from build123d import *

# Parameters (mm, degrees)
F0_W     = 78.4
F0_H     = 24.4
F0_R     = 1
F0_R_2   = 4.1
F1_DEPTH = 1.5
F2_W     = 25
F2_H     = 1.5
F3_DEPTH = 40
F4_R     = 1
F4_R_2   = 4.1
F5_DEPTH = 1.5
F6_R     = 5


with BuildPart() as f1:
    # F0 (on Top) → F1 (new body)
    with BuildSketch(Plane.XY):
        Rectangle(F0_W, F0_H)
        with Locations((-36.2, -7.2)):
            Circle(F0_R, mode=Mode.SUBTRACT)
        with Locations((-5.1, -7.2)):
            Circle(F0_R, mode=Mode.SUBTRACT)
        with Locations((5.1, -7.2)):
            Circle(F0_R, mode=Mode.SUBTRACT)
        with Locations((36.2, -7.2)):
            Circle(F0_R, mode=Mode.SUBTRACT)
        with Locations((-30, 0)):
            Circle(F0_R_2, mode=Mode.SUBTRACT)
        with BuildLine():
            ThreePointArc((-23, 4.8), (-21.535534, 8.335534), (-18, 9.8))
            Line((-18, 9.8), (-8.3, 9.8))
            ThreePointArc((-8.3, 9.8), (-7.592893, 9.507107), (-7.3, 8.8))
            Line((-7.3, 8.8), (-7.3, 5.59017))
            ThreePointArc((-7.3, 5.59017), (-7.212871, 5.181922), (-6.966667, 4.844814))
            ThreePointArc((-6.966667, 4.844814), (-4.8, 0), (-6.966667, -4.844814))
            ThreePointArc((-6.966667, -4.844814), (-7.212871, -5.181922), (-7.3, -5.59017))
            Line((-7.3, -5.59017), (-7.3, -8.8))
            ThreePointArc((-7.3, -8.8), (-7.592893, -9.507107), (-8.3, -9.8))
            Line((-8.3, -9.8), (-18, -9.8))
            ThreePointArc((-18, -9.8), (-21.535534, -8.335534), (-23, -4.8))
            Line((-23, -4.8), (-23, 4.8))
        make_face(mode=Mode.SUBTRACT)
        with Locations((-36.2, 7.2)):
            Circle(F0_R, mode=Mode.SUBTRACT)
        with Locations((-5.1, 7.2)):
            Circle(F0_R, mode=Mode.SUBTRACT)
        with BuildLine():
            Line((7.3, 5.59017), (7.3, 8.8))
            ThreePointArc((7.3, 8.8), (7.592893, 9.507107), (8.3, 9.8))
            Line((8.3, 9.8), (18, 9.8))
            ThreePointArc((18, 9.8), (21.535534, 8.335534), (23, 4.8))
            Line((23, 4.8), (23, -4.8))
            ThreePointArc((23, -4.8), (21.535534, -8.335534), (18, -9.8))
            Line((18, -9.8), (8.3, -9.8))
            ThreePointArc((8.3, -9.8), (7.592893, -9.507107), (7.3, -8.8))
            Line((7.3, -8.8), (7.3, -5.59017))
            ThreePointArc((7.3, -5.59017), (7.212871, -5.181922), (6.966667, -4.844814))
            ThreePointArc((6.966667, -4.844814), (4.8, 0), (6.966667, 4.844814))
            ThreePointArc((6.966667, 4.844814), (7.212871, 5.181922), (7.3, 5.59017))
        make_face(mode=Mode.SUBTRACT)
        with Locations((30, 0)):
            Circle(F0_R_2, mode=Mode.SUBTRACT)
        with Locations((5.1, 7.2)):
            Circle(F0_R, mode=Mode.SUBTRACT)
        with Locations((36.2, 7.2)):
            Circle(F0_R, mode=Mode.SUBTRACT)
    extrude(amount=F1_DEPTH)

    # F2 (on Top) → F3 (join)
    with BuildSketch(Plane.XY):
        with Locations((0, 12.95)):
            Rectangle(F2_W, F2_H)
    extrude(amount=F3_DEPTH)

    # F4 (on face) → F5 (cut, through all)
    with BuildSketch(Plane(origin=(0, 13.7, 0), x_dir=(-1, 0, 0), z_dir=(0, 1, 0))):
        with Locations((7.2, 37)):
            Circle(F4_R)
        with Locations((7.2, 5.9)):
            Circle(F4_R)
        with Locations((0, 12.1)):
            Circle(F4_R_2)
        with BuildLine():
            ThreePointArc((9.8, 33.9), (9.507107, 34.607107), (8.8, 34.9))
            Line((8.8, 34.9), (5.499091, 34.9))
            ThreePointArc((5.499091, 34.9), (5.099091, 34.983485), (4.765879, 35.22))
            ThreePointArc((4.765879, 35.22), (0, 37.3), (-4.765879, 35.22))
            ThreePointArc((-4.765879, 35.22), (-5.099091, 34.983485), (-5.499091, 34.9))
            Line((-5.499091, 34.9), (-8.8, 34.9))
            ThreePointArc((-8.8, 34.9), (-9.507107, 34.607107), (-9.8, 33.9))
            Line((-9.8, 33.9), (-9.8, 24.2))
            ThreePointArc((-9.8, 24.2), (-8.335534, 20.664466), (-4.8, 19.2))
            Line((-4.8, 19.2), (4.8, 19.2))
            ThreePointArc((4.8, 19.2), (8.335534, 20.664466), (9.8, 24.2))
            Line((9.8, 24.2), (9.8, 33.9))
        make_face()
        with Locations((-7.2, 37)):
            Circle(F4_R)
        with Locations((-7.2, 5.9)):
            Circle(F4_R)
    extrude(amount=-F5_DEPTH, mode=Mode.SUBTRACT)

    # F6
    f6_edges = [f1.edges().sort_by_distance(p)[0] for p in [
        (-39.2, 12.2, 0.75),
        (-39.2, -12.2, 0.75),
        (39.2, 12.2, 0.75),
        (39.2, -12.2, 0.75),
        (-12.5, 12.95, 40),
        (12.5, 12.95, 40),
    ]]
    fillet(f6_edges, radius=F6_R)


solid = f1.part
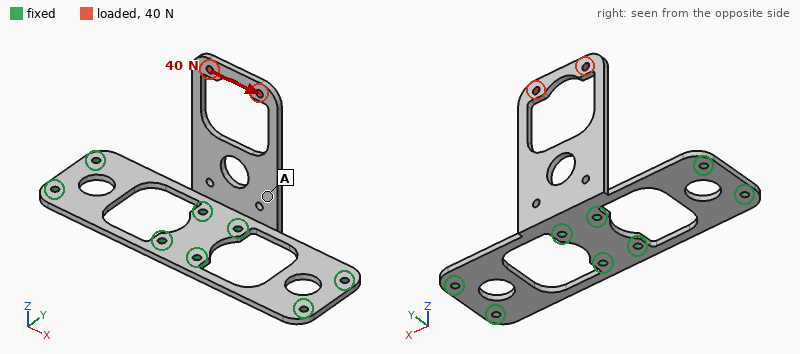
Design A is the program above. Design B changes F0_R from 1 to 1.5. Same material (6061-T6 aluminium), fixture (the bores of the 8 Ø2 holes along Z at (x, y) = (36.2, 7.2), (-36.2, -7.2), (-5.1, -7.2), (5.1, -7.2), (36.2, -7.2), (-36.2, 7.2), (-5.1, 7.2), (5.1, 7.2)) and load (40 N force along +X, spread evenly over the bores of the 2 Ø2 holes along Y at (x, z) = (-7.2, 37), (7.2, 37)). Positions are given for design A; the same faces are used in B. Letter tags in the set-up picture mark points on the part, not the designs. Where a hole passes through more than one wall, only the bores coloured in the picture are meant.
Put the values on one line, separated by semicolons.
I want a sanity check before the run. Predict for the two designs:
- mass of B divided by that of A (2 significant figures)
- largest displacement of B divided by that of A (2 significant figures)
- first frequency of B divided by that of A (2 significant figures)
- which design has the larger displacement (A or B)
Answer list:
0.98; 0.85; 1.0; A
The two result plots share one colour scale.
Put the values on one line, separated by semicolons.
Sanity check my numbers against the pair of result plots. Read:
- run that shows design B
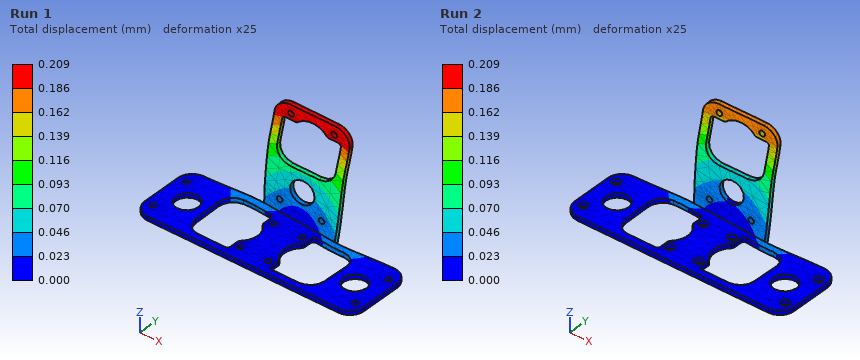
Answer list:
Run 2
